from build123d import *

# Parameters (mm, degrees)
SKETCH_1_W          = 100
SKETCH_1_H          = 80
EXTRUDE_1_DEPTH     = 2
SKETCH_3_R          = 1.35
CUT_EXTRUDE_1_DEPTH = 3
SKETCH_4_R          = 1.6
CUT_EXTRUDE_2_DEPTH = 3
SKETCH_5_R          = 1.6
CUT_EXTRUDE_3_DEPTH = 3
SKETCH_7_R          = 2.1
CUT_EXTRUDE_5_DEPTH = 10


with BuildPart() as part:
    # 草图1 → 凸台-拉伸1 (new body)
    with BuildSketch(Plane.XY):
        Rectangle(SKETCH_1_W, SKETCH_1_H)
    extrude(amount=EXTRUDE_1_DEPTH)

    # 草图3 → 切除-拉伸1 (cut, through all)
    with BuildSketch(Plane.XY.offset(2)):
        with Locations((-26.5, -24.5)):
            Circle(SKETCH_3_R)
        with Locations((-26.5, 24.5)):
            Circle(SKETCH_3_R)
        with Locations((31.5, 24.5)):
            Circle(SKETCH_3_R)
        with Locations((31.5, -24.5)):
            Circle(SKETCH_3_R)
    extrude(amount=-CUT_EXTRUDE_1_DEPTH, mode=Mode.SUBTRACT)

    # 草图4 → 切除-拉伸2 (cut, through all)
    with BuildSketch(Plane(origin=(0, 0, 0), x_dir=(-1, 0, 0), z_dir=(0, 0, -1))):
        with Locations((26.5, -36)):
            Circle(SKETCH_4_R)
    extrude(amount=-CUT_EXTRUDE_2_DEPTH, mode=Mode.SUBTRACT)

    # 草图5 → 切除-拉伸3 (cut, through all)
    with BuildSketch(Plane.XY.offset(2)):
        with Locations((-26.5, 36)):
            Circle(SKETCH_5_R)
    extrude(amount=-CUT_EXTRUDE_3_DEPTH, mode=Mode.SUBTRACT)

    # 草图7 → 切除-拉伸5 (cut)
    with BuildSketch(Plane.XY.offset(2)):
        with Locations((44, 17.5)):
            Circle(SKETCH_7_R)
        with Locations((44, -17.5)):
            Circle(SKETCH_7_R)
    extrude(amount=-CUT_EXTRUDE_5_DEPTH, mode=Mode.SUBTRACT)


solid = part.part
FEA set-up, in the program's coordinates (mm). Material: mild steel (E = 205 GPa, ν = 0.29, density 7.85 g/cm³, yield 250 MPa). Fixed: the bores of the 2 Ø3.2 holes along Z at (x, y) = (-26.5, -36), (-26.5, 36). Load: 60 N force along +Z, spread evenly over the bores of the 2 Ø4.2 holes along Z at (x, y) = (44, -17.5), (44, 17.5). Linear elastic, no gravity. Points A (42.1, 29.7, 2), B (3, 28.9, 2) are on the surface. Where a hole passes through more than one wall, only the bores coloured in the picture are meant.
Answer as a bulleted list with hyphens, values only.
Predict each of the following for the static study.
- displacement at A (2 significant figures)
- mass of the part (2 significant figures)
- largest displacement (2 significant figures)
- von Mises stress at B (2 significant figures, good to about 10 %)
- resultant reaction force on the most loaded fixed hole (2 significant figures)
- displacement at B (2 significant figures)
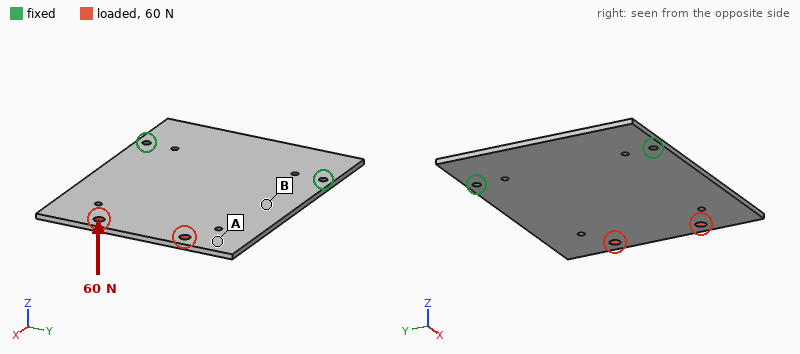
- 0.85 mm
- 120 g
- 1.0 mm
- 47 MPa
- 30 N
- 0.24 mm
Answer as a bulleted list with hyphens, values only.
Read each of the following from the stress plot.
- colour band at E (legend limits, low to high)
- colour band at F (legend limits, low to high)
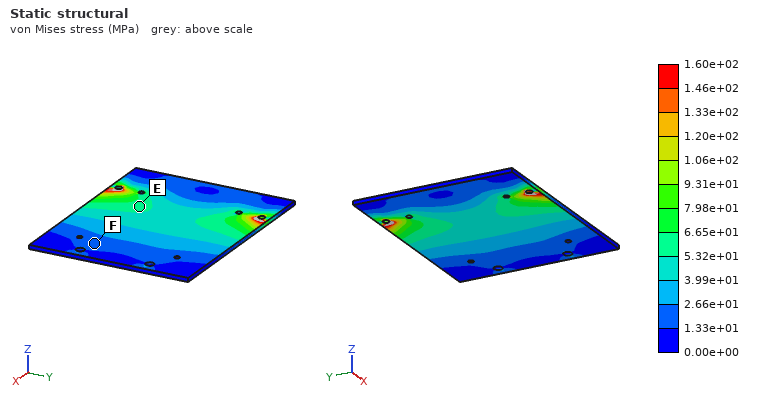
- 5.32e+01 to 6.65e+01 MPa
- 1.33e+01 to 2.66e+01 MPa
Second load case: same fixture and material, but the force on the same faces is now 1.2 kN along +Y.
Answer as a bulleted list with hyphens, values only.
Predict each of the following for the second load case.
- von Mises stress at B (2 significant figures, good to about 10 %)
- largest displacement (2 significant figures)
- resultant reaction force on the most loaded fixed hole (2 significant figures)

- 20 MPa
- 21 µm
- 1.3 kN
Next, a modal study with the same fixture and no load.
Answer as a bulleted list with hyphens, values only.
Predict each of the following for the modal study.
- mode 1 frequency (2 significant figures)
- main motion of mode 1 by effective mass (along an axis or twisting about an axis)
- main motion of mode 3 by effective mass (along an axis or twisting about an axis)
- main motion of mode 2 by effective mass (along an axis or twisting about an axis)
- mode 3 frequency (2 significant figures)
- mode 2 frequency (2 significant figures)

- 230 Hz
- along Z
- along Z
- twisting about X
- 1500 Hz
- 680 Hz
